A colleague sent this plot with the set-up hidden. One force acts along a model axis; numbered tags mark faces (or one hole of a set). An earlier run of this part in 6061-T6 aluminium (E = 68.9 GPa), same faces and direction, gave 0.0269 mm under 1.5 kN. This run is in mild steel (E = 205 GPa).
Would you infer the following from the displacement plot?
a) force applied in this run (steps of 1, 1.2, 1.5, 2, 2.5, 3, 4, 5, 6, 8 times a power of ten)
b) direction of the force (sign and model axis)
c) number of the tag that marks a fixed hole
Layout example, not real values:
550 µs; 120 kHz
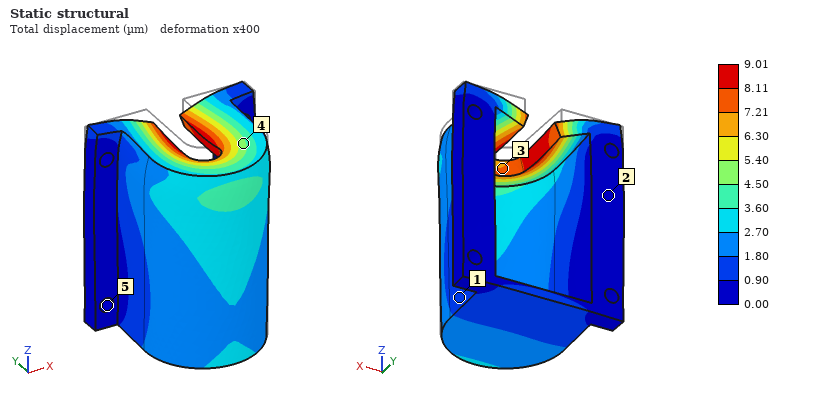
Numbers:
1.5 kN; -Z; 5
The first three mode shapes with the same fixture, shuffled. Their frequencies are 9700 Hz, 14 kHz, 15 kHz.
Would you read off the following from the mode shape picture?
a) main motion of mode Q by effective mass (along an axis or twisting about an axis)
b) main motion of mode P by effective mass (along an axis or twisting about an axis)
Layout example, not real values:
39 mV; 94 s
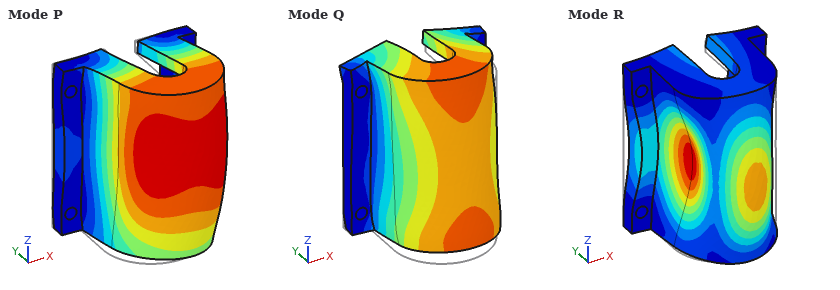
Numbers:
along Z; along X
